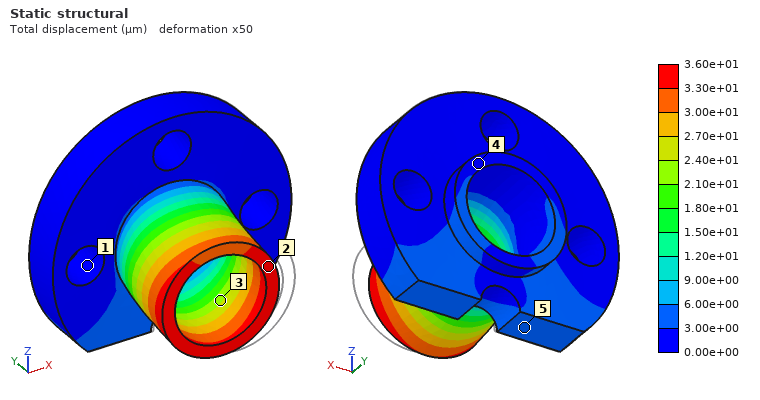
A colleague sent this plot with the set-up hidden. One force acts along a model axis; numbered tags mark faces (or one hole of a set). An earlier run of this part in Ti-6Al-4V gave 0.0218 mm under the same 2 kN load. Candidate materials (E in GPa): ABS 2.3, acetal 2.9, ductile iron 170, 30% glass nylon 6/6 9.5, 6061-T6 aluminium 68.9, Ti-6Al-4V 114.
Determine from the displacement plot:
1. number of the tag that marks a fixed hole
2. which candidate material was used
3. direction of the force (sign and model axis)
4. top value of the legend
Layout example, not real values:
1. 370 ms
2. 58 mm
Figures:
1. 1
2. 6061-T6 aluminium
3. -X
4. 3.60e+01 µm
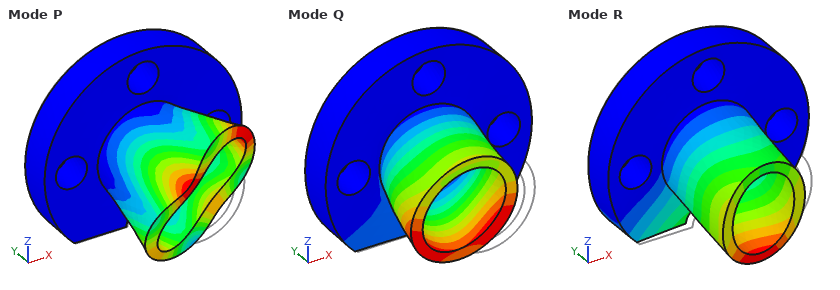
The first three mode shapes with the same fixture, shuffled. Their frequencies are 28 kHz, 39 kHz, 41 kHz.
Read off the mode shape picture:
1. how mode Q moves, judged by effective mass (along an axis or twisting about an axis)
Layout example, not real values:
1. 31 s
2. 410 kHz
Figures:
1. along X
